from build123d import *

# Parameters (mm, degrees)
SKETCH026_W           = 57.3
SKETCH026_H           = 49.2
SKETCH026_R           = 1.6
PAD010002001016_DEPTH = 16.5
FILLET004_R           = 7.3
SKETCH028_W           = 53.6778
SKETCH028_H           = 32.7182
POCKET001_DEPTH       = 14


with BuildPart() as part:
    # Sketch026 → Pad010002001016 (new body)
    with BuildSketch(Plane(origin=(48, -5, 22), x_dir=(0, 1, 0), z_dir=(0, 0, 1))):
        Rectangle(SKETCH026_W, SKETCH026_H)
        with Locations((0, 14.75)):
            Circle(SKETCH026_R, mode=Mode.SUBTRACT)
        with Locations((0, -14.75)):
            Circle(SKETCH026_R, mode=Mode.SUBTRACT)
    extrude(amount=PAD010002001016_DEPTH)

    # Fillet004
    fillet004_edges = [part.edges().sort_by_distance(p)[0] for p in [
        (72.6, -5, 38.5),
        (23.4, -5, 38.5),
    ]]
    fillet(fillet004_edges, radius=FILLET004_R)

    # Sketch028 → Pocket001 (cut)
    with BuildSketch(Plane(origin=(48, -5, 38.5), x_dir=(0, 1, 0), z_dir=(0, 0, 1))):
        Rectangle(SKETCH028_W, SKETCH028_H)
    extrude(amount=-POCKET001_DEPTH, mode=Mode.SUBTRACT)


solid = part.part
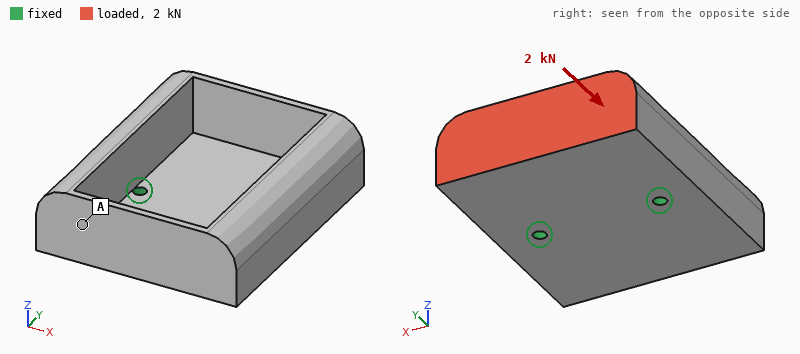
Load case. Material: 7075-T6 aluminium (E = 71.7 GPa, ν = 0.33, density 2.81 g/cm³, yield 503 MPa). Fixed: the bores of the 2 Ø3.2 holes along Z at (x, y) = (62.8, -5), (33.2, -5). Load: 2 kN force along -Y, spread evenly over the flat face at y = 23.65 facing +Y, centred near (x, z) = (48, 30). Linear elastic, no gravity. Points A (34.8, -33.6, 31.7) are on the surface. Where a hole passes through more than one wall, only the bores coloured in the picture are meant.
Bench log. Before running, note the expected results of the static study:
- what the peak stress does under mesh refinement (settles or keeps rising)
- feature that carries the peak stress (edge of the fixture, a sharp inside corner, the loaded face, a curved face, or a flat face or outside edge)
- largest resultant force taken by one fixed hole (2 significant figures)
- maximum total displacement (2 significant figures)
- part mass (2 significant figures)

keeps rising
edge of the fixture
1.0 kN
0.32 mm
58 g
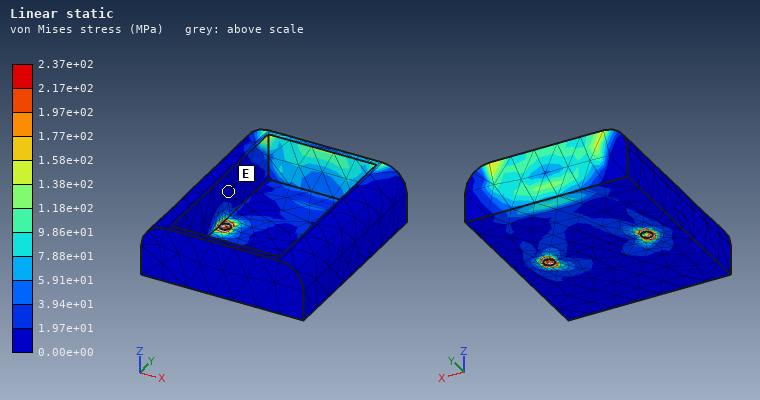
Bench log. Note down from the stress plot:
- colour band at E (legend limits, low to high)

0.00e+00 to 1.97e+01 MPa
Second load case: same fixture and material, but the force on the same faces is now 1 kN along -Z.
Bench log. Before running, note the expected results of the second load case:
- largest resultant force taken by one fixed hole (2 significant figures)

520 N
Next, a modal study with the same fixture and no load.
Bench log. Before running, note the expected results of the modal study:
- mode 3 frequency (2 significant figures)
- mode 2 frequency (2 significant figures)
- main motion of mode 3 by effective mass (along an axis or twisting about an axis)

5600 Hz
4500 Hz
along X
